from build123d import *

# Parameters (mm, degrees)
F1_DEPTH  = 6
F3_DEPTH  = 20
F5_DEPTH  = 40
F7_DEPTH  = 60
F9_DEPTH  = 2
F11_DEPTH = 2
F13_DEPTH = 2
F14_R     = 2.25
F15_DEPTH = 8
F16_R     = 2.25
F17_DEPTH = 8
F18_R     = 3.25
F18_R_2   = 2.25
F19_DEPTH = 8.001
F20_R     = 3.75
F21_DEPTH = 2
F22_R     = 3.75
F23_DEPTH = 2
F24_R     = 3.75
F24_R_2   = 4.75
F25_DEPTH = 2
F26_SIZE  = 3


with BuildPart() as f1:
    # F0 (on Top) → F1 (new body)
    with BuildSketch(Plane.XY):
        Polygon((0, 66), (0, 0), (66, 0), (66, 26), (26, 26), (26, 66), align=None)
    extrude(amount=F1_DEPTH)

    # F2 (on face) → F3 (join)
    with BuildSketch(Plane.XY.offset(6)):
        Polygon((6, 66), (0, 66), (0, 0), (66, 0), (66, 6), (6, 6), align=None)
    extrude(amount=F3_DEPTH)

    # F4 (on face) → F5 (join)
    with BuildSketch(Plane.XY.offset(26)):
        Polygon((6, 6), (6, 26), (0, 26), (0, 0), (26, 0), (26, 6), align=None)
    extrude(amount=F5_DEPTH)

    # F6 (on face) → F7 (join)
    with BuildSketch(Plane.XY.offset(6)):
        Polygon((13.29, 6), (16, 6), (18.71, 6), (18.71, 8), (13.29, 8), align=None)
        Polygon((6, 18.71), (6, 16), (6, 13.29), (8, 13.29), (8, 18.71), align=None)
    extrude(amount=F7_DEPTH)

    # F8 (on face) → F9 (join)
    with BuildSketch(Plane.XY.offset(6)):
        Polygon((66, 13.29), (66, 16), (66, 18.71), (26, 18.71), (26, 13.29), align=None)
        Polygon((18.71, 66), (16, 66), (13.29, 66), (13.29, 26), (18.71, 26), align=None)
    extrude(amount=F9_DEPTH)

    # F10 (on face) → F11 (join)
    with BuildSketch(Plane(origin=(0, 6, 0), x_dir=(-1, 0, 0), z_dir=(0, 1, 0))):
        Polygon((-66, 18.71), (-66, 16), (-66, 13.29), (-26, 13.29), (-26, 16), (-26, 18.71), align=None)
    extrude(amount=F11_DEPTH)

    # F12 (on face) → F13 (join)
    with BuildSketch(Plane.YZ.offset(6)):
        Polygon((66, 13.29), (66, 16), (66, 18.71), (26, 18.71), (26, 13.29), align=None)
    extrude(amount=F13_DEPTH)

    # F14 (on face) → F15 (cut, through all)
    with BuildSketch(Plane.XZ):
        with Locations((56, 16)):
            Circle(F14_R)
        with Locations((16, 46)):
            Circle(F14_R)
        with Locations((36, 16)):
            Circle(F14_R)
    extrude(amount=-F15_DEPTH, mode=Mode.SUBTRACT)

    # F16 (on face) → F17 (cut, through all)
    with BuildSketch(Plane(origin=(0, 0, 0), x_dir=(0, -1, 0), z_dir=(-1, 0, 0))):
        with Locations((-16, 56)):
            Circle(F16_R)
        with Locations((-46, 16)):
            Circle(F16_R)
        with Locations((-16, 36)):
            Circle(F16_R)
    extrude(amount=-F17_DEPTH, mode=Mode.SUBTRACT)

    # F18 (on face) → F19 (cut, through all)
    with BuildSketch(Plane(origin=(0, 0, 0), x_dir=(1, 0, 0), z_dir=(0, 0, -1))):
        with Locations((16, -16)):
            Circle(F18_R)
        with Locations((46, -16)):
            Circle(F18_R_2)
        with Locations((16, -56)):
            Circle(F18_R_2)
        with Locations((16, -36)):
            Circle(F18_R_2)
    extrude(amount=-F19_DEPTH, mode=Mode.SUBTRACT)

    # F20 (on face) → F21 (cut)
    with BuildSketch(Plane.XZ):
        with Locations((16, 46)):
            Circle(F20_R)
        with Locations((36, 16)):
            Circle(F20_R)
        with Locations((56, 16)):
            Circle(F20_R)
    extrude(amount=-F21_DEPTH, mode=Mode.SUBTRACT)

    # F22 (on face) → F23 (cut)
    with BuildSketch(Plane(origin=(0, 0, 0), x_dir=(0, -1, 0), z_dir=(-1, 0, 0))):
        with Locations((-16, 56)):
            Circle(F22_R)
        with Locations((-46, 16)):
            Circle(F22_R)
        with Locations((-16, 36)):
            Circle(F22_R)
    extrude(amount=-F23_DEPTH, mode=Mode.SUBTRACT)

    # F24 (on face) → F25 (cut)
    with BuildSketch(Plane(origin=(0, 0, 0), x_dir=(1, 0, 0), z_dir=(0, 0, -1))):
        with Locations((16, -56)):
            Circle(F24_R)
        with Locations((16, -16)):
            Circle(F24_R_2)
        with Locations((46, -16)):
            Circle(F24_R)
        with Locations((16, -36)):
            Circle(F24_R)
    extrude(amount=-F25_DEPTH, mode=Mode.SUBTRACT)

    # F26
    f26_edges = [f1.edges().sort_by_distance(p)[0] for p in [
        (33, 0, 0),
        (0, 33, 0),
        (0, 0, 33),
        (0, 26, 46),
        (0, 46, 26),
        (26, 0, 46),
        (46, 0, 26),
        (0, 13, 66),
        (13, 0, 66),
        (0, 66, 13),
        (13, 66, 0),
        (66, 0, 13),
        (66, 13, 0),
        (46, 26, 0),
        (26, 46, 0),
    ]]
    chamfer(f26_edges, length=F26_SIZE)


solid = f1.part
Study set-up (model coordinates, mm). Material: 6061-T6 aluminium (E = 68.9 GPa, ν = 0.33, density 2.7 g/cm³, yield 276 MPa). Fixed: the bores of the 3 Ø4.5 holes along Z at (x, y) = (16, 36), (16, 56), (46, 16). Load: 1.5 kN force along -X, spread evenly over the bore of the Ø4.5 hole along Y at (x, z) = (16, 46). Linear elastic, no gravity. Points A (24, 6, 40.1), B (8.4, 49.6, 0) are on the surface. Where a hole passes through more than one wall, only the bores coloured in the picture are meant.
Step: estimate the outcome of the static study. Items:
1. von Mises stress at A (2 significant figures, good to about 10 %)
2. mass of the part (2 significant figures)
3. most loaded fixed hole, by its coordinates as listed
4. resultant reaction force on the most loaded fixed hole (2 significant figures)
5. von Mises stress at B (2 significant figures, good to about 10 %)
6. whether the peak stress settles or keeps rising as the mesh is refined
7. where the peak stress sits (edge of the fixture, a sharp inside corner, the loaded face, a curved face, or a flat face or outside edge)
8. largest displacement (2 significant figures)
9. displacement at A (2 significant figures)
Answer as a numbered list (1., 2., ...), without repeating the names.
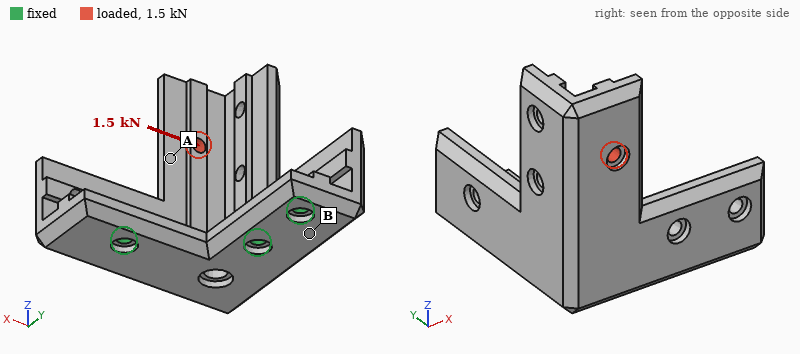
1. 21 MPa
2. 110 g
3. (16, 36)
4. 2.3 kN
5. 50 MPa
6. keeps rising
7. edge of the fixture
8. 0.41 mm
9. 0.21 mm
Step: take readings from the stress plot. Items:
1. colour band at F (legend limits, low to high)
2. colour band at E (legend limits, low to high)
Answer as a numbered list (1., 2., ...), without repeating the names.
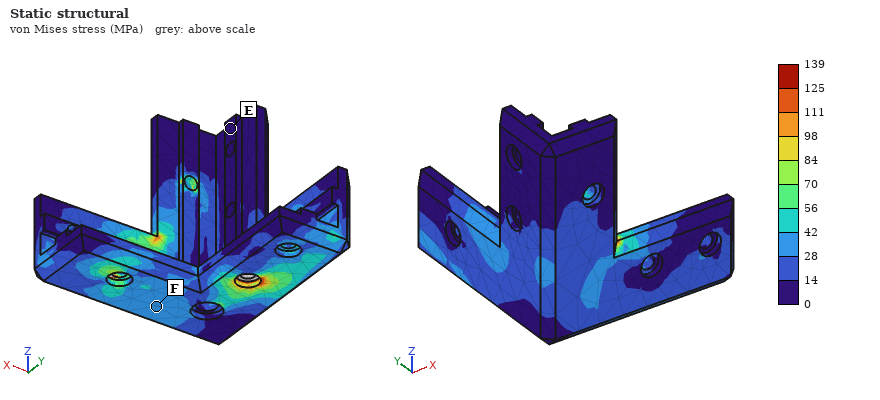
1. 28 to 42 MPa
2. 0 to 14 MPa
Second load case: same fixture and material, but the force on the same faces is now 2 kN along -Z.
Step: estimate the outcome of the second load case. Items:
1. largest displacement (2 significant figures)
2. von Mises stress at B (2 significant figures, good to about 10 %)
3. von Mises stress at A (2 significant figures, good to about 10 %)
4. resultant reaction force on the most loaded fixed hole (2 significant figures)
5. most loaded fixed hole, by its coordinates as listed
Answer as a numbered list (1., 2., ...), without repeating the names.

1. 0.31 mm
2. 48 MPa
3. 21 MPa
4. 2.4 kN
5. (16, 36)
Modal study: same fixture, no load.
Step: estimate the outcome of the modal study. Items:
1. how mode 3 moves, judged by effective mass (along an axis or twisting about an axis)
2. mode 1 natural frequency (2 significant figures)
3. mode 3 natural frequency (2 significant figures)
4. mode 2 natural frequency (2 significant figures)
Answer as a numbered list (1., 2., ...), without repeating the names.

1. along Z
2. 1600 Hz
3. 4900 Hz
4. 2900 Hz
